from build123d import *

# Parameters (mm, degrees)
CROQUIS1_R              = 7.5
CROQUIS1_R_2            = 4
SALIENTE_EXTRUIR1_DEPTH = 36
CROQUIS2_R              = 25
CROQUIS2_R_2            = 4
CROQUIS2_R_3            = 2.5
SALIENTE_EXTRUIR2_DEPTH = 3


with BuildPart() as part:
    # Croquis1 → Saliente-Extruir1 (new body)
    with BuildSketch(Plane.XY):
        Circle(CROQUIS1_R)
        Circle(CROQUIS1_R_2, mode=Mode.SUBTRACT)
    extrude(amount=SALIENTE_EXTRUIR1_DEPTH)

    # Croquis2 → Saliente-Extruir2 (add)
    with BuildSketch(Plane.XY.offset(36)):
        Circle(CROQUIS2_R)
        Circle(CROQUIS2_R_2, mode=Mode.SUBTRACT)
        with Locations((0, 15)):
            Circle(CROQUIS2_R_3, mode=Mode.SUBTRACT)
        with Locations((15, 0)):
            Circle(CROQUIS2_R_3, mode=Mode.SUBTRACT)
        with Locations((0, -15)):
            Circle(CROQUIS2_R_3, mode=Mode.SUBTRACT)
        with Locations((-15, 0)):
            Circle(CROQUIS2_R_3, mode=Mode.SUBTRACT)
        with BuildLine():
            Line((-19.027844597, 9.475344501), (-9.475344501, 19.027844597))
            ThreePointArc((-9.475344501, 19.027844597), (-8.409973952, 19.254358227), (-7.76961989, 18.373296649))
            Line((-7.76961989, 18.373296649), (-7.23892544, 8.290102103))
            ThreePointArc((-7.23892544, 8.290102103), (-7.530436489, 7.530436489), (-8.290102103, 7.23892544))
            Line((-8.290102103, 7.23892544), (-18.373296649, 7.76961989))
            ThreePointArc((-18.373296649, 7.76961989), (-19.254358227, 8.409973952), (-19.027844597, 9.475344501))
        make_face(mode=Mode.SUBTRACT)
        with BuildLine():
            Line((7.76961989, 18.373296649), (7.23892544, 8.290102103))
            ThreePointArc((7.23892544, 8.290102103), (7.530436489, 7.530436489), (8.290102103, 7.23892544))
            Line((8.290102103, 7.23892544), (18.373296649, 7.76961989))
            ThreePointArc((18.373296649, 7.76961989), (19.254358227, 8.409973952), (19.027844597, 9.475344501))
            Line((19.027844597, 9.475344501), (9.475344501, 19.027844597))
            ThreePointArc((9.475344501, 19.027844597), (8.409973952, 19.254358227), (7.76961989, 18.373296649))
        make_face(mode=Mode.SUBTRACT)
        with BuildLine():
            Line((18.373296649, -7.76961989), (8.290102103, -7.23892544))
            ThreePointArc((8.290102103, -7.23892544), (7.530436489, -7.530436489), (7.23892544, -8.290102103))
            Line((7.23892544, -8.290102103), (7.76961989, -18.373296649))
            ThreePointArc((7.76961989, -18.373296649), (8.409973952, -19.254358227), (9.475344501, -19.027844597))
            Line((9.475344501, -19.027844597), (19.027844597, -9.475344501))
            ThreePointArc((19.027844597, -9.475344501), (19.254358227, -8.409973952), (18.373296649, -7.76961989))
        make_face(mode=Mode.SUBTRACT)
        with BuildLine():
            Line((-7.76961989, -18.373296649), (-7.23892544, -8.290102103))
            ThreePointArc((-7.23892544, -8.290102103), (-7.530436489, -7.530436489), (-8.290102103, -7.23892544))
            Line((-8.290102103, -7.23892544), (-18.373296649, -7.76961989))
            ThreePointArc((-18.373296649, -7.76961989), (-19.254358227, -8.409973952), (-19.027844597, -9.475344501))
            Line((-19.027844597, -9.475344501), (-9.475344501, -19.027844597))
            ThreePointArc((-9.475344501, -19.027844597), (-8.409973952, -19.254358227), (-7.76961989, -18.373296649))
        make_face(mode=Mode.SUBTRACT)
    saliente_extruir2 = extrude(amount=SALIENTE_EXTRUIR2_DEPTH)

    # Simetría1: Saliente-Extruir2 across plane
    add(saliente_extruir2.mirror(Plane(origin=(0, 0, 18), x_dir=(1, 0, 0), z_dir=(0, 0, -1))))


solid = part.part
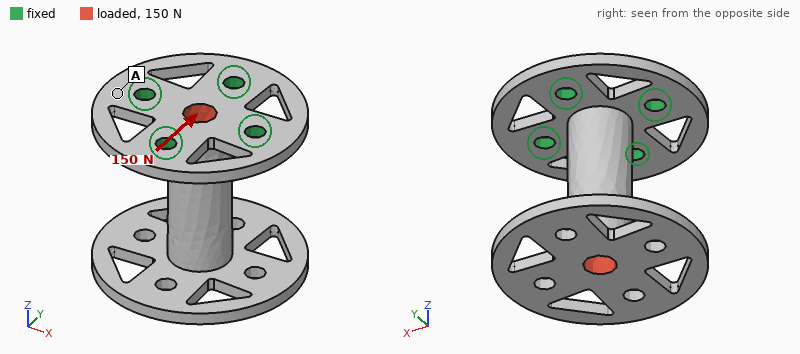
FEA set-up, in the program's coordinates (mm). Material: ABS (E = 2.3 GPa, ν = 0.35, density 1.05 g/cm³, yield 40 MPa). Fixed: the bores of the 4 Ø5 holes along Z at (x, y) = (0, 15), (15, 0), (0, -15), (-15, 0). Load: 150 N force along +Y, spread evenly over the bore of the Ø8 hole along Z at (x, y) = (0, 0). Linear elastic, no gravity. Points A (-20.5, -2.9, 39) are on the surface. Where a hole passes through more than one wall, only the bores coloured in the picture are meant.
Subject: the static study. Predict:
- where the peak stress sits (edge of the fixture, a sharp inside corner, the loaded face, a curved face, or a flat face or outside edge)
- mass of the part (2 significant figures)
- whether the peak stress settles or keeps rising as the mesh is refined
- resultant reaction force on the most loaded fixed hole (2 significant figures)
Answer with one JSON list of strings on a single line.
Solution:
["edge of the fixture", "14 g", "keeps rising", "140 N"]
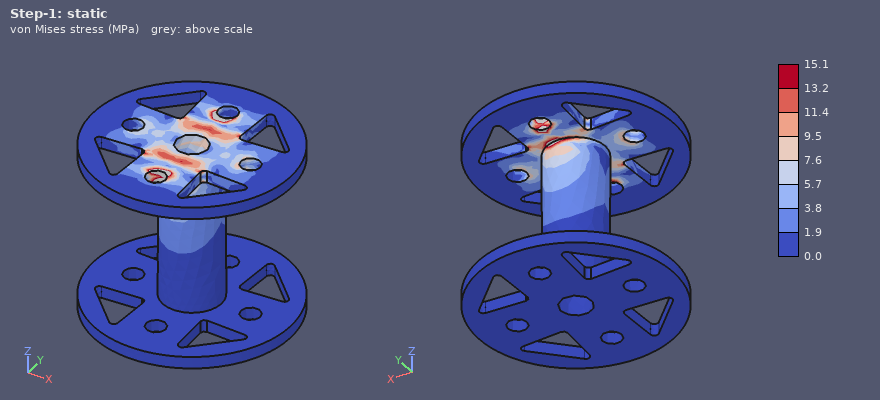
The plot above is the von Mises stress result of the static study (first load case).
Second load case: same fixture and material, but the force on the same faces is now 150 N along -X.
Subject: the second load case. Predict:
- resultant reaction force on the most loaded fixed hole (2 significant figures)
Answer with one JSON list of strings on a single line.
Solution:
["140 N"]
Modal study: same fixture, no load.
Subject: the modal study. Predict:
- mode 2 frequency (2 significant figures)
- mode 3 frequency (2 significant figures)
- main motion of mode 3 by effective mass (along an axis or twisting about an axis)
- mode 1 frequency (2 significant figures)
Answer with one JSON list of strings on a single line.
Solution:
["620 Hz", "1200 Hz", "twisting about Z", "620 Hz"]
